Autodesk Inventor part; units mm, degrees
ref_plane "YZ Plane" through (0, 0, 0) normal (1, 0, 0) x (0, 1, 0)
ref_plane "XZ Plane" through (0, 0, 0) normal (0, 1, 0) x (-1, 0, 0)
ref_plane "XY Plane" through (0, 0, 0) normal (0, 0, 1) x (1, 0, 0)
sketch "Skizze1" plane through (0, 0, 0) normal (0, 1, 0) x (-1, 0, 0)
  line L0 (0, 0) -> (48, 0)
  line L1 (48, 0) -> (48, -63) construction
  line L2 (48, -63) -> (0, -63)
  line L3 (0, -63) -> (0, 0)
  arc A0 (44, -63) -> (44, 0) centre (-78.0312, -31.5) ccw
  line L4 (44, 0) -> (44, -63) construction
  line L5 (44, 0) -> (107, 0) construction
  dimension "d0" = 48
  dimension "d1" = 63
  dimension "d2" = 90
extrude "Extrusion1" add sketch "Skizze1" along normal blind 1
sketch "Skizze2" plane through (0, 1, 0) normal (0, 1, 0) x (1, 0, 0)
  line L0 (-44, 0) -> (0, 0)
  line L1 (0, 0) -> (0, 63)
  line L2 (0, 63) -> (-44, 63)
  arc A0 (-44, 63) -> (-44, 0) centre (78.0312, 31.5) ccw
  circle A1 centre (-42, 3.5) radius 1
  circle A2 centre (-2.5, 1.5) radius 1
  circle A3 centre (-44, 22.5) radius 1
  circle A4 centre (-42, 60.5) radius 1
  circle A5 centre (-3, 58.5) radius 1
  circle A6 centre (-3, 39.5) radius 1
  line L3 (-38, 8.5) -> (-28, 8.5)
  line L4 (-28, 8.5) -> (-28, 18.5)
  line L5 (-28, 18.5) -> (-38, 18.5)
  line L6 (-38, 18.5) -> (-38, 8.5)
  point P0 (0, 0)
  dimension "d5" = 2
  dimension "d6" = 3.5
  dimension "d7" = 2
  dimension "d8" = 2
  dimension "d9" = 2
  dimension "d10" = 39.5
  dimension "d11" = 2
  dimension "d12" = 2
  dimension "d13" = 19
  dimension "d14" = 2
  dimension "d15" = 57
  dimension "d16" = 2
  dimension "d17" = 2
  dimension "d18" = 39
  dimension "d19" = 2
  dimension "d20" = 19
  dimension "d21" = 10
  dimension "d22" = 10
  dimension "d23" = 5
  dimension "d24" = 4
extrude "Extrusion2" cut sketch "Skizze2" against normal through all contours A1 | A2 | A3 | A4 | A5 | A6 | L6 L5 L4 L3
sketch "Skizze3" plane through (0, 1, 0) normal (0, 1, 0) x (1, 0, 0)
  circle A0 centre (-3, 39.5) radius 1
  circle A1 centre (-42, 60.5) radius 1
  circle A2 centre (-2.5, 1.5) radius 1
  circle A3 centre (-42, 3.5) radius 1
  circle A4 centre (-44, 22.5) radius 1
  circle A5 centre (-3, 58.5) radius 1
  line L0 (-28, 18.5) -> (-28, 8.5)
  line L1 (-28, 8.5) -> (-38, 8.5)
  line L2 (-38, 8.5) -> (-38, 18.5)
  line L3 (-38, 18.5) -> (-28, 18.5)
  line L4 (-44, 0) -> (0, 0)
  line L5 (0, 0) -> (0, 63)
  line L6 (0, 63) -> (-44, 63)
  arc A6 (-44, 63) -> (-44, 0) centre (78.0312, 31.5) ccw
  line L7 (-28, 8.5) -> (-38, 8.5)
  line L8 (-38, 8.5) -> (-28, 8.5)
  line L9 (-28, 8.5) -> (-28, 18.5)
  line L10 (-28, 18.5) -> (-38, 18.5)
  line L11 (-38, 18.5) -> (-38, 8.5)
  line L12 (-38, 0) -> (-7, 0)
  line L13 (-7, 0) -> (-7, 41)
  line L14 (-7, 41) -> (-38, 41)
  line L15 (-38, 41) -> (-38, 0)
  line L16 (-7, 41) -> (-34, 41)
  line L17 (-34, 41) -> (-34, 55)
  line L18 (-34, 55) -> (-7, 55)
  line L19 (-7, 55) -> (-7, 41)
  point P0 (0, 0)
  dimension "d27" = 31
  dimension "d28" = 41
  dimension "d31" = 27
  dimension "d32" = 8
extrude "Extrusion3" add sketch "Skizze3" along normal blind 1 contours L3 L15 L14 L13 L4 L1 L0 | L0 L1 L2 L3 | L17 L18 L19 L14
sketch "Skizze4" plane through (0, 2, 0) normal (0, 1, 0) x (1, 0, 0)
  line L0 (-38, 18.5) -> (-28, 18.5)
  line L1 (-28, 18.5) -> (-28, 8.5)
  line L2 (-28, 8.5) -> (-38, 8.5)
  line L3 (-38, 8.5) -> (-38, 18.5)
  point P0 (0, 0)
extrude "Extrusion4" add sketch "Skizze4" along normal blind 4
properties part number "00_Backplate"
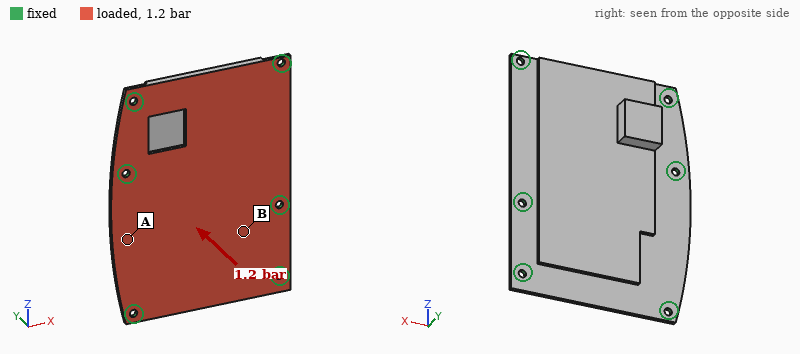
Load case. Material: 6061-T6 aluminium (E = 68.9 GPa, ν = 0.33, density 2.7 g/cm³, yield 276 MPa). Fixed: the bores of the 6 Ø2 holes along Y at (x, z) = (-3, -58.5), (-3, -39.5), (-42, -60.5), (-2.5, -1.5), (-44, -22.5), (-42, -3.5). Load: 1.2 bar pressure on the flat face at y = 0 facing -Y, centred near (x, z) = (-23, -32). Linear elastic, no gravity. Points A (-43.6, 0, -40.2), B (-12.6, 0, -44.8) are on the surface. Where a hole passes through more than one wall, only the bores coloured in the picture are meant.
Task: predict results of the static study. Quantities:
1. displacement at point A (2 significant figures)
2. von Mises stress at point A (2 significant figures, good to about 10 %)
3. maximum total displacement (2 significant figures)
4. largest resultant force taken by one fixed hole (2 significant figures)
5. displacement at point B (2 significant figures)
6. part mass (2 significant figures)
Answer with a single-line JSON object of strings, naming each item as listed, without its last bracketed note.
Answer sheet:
{"displacement at point A": "90 µm", "von Mises stress at point A": "27 MPa", "maximum total displacement": "93 µm", "largest resultant force taken by one fixed hole": "170 N", "displacement at point B": "45 µm", "part mass": "13 g"}
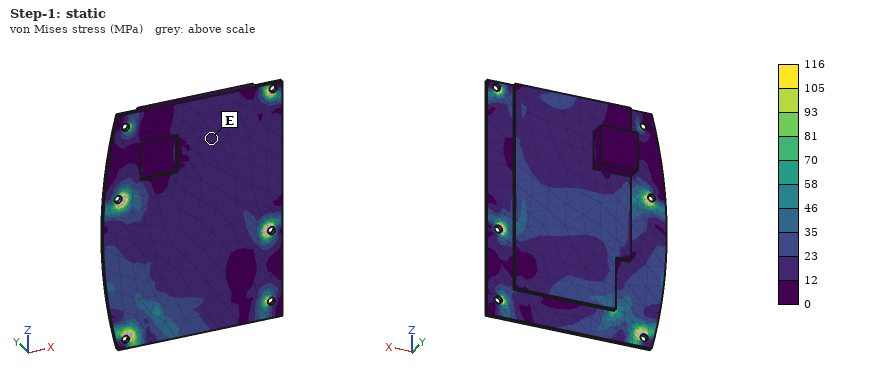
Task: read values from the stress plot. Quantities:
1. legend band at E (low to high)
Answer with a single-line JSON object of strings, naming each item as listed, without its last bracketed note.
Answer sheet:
{"legend band at E": "12 to 23 MPa"}
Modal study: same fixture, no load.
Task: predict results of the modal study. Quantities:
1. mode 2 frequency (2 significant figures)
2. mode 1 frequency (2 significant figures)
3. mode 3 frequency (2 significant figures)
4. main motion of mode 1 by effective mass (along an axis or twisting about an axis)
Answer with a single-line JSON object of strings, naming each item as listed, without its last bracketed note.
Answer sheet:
{"mode 2 frequency": "4000 Hz", "mode 1 frequency": "3100 Hz", "mode 3 frequency": "5400 Hz", "main motion of mode 1 by effective mass": "along Y"}
